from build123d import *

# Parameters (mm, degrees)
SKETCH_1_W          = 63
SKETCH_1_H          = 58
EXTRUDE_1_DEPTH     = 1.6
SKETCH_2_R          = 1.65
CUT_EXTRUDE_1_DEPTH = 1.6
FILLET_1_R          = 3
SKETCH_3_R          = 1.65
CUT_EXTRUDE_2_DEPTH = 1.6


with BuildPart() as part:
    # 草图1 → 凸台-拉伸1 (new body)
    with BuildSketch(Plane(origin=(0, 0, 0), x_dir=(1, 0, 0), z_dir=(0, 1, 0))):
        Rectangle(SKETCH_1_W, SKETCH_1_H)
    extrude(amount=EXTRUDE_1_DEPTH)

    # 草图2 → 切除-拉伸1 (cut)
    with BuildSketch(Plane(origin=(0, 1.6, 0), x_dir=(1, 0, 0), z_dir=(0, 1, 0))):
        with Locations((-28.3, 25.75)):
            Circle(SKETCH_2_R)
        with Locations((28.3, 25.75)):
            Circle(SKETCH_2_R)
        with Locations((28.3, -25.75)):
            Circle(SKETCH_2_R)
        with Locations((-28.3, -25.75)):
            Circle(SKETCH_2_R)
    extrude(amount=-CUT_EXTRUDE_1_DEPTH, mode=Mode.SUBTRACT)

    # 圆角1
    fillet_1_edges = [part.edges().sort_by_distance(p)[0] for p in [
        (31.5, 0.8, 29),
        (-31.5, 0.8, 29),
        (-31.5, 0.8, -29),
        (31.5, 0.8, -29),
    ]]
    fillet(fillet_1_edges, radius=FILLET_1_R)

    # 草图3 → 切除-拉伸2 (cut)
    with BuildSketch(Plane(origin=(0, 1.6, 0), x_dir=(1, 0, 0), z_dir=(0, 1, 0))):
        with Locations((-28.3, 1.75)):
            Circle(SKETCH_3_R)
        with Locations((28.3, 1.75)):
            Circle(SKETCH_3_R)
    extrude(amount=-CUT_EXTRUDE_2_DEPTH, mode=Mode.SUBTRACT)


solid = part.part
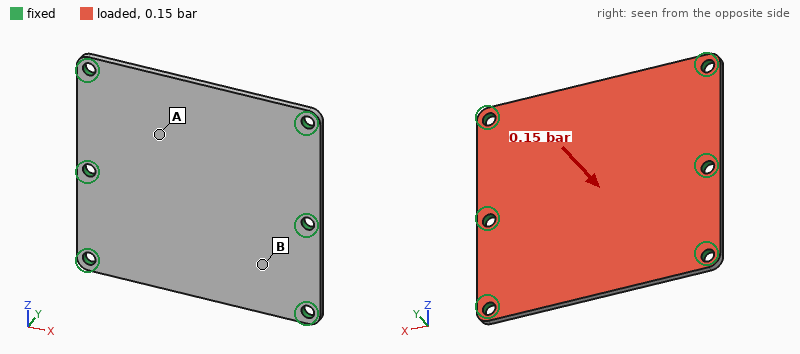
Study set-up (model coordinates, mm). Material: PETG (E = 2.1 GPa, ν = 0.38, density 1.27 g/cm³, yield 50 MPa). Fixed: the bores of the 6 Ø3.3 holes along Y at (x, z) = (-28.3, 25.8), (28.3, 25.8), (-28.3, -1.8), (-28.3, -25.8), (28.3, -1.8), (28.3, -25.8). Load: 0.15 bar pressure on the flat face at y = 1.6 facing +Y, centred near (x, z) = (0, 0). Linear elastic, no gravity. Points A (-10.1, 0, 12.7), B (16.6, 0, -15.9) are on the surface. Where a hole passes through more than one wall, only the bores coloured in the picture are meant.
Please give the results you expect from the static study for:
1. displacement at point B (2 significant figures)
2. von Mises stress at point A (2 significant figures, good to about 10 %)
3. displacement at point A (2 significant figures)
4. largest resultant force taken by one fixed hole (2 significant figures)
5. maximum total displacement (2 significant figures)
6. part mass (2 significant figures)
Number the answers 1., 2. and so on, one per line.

1. 0.27 mm
2. 2.8 MPa
3. 0.47 mm
4. 12 N
5. 0.62 mm
6. 7.3 g
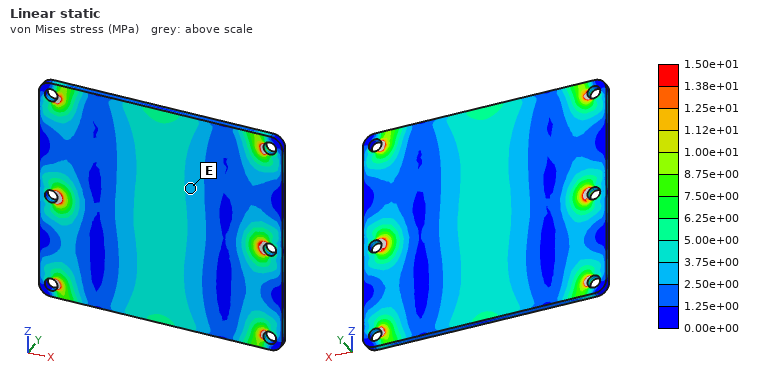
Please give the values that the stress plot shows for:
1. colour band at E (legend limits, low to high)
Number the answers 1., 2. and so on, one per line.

1. 2.50e+00 to 3.75e+00 MPa
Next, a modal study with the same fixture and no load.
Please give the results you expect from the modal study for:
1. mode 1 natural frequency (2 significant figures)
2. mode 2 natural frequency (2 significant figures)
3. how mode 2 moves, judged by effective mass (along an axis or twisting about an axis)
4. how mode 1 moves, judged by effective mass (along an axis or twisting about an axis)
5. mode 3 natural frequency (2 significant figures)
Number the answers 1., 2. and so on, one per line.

1. 650 Hz
2. 800 Hz
3. twisting about X
4. along Y
5. 1300 Hz
